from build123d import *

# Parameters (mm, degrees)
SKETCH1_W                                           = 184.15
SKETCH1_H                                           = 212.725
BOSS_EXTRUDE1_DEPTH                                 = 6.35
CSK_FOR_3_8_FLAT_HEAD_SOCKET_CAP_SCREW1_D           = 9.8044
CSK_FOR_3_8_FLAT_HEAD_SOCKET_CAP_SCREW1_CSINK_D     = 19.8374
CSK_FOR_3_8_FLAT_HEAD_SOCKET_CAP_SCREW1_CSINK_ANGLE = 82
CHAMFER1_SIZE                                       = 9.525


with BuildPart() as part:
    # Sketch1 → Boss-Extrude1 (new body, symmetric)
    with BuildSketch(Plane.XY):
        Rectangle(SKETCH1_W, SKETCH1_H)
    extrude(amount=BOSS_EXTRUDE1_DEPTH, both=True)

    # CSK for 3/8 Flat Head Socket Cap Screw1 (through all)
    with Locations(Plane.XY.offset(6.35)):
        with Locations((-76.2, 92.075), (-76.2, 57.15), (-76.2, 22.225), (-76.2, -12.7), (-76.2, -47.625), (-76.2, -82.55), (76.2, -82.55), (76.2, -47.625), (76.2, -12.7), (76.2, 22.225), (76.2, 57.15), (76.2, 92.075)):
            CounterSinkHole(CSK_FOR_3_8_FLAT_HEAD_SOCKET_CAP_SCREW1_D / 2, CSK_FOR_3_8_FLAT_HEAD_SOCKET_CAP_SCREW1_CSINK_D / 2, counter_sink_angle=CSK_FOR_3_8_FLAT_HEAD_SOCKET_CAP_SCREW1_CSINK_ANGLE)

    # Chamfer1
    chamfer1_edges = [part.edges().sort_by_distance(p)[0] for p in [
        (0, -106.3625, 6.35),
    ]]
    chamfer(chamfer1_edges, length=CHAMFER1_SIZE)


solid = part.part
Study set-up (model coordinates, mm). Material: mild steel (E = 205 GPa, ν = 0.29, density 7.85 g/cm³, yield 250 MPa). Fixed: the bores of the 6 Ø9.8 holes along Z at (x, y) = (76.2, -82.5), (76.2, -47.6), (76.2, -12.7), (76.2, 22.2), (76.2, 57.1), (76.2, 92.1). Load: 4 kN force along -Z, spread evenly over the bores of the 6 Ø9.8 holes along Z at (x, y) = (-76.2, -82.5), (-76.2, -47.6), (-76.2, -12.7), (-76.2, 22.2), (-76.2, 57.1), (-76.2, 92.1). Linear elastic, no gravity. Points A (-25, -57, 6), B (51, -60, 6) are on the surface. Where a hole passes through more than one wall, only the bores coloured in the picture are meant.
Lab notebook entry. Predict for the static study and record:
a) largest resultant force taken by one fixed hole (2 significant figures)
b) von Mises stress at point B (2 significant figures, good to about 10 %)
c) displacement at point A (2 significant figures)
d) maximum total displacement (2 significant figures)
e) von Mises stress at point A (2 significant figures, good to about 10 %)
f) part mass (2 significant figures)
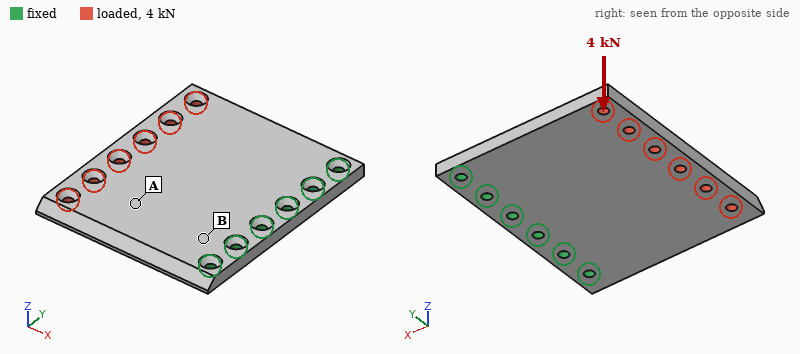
1.4 kN
85 MPa
0.39 mm
0.85 mm
36 MPa
3.7 kg
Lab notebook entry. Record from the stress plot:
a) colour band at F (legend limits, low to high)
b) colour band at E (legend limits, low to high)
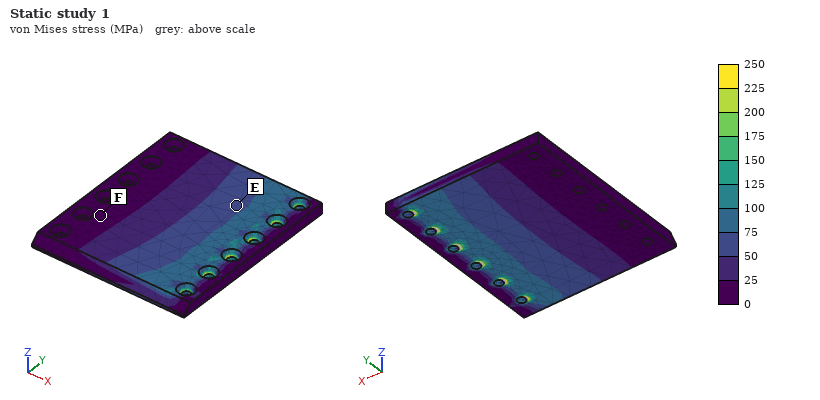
0 to 25 MPa
50 to 75 MPa
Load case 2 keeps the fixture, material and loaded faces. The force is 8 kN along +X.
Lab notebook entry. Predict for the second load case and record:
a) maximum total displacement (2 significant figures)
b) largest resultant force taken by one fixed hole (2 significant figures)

42 µm
1.5 kN
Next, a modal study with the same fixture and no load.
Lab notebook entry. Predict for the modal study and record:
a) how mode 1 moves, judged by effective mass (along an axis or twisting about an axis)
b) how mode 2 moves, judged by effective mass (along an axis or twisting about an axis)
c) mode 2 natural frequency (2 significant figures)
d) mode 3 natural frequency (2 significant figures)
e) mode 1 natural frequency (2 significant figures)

along Z
twisting about X
750 Hz
1900 Hz
350 Hz
